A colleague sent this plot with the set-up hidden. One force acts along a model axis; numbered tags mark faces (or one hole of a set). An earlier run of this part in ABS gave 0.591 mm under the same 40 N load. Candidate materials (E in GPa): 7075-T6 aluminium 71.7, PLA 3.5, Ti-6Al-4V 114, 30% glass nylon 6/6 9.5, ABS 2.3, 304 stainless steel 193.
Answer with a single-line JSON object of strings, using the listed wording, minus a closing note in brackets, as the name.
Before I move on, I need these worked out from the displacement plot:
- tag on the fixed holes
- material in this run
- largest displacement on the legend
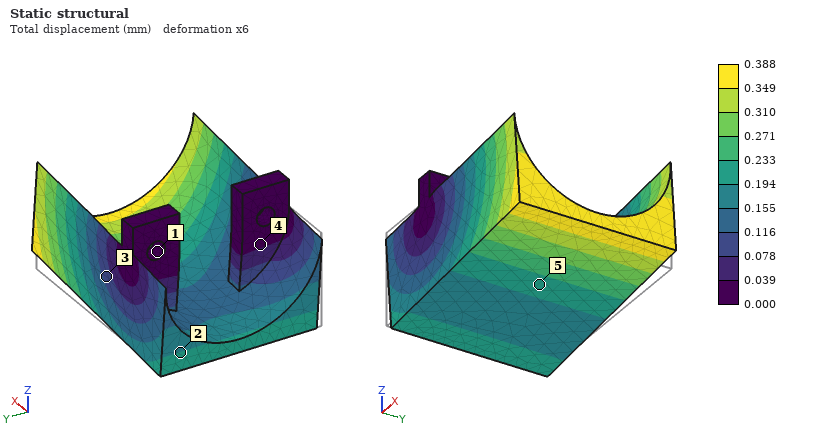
{"tag on the fixed holes": "1", "material in this run": "PLA", "largest displacement on the legend": "0.388 mm"}
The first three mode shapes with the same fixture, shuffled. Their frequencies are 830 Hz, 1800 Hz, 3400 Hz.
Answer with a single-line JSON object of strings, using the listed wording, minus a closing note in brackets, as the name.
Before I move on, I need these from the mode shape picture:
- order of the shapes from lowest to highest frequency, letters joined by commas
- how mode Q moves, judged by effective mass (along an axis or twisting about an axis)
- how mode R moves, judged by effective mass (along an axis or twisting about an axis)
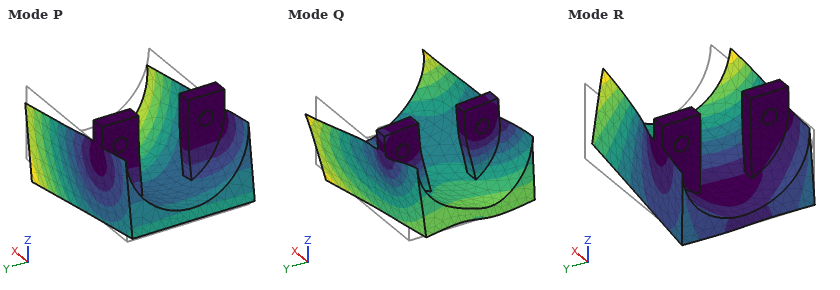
{"order of the shapes from lowest to highest frequency, letters joined by commas": "P, R, Q", "how mode Q moves, judged by effective mass": "along Y", "how mode R moves, judged by effective mass": "along Y"}
